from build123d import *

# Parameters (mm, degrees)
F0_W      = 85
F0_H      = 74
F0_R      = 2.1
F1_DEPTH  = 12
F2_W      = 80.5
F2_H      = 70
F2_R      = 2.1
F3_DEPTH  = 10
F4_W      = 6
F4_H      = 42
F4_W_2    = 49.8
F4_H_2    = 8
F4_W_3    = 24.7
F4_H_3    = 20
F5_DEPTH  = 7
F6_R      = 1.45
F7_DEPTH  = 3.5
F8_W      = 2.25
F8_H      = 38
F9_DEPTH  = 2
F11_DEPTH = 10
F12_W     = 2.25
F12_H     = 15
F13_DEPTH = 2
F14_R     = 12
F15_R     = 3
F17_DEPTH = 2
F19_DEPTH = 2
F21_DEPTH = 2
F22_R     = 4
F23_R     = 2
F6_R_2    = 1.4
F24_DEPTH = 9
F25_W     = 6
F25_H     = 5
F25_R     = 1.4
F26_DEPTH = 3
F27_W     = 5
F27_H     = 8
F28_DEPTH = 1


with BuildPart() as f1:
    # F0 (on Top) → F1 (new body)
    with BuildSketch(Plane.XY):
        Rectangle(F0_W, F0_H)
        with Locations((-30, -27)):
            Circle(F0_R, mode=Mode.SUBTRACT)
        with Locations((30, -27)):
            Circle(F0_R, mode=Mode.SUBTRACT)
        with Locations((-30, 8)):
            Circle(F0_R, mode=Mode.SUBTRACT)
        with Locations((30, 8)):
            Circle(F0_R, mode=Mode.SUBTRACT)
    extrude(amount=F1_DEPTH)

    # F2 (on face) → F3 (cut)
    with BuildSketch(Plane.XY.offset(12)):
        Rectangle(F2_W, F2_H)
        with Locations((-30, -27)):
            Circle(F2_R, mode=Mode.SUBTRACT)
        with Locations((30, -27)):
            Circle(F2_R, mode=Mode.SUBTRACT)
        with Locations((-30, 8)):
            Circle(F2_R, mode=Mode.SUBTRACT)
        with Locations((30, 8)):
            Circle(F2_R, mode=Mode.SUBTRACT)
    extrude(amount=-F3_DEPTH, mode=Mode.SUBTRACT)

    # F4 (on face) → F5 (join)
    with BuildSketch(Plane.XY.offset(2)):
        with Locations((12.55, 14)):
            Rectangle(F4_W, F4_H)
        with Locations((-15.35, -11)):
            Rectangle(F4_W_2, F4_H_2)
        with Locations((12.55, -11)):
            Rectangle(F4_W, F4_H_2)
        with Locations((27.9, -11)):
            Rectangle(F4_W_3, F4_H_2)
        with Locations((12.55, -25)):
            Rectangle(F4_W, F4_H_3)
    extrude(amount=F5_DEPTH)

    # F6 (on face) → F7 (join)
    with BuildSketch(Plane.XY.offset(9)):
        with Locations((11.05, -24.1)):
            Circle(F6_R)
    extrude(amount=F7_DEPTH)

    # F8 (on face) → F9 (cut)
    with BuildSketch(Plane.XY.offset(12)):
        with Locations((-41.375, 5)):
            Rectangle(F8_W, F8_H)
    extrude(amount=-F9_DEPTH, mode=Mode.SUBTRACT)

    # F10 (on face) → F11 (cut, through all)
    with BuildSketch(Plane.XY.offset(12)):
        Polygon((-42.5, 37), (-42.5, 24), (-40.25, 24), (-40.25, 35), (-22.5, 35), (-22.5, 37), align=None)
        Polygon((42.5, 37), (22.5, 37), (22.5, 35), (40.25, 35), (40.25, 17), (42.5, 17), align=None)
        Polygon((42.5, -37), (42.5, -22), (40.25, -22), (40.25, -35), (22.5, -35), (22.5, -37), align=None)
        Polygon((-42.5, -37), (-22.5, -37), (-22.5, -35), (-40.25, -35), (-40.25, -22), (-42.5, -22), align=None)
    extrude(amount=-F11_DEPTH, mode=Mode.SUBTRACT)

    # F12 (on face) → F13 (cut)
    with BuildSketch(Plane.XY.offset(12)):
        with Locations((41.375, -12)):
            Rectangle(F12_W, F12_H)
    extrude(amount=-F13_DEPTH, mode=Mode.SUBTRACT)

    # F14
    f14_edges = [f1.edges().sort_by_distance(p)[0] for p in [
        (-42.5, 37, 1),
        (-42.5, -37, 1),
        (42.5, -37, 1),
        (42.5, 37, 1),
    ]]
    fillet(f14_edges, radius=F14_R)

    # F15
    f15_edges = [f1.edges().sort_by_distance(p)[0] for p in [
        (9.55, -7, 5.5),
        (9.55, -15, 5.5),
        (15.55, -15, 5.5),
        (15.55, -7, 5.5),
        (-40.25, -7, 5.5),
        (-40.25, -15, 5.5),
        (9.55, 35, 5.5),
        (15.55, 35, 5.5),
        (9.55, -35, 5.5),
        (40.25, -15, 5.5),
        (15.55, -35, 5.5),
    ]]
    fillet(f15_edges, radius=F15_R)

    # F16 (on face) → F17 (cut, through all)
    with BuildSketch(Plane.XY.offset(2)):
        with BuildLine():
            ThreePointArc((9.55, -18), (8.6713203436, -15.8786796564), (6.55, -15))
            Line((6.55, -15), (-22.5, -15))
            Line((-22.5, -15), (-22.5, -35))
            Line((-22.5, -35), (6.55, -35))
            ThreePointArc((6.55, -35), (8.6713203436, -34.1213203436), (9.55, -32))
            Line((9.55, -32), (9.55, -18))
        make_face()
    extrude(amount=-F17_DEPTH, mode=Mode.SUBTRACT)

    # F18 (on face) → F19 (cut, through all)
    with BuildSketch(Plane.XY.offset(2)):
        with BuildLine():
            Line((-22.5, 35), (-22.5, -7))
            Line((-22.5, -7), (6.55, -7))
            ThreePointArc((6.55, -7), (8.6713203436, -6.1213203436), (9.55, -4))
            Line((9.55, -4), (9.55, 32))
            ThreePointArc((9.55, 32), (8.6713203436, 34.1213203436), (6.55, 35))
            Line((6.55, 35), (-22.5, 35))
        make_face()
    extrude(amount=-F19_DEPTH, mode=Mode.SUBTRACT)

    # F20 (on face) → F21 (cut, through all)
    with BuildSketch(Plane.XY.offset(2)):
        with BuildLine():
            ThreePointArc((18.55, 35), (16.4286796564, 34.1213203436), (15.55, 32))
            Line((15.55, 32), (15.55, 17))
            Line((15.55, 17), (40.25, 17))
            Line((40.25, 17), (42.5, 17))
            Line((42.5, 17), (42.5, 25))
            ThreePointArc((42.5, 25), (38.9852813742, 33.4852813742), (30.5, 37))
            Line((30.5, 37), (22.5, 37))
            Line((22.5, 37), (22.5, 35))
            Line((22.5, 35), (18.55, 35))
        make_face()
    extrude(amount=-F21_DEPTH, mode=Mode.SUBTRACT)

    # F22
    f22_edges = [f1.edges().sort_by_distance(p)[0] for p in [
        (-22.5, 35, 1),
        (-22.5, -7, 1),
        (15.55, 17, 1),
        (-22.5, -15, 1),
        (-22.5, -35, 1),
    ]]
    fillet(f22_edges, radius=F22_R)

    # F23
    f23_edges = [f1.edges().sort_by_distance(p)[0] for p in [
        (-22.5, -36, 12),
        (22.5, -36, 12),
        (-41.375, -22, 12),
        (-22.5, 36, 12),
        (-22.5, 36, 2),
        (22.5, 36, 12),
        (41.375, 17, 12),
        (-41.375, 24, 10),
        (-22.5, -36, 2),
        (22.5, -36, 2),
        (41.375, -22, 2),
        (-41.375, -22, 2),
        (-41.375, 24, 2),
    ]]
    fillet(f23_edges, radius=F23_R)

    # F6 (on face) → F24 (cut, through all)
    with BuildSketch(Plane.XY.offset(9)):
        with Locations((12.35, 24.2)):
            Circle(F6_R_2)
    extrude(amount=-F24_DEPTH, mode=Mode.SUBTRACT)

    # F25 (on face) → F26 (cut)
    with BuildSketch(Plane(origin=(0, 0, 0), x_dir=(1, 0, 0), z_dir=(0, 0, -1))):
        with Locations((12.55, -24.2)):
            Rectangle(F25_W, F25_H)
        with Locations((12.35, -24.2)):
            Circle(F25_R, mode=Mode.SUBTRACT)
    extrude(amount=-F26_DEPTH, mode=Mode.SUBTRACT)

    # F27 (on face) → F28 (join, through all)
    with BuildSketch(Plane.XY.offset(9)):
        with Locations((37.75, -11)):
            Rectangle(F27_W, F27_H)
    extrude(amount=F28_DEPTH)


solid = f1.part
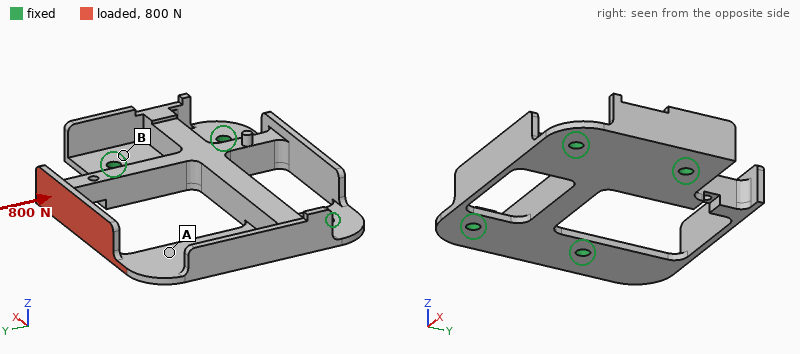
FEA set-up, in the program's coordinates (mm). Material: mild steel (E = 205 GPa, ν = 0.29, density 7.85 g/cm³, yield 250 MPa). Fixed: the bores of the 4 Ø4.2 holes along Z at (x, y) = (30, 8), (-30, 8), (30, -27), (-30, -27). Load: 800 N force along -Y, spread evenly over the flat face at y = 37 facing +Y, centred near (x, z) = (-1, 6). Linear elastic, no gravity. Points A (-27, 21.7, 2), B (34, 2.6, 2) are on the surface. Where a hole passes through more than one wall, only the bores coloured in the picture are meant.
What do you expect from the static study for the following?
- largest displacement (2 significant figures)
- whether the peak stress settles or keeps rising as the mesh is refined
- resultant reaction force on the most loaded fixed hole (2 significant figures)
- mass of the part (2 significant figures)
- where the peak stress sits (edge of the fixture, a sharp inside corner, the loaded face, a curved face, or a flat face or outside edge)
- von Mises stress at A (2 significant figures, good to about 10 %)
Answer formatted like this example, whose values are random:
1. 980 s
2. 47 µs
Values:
1. 0.12 mm
2. keeps rising
3. 310 N
4. 140 g
5. a sharp inside corner
6. 42 MPa
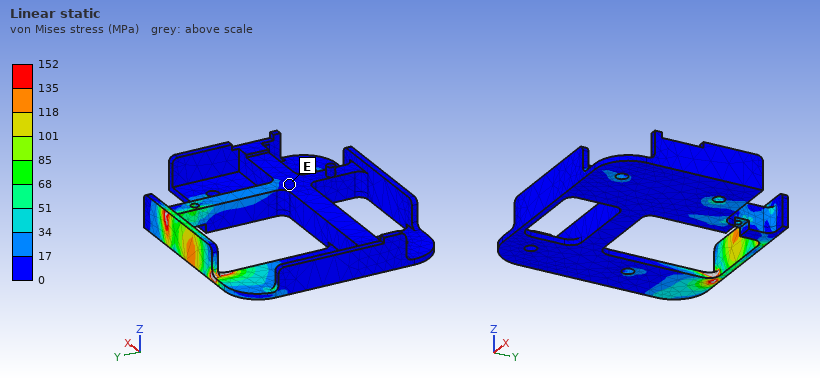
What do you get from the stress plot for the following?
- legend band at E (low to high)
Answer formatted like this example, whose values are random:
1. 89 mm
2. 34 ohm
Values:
1. 0 to 17 MPa
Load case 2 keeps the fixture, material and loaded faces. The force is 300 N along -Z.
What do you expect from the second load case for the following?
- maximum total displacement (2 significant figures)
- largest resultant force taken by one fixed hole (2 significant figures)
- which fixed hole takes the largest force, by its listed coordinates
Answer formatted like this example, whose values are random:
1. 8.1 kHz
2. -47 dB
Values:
1. 0.16 mm
2. 340 N
3. (30, 8)
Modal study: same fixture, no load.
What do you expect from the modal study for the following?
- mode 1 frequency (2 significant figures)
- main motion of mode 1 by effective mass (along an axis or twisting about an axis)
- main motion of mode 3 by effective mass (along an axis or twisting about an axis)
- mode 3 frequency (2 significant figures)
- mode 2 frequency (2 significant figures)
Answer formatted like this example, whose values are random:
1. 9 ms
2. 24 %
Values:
1. 2100 Hz
2. along Z
3. along Z
4. 4600 Hz
5. 3600 Hz
